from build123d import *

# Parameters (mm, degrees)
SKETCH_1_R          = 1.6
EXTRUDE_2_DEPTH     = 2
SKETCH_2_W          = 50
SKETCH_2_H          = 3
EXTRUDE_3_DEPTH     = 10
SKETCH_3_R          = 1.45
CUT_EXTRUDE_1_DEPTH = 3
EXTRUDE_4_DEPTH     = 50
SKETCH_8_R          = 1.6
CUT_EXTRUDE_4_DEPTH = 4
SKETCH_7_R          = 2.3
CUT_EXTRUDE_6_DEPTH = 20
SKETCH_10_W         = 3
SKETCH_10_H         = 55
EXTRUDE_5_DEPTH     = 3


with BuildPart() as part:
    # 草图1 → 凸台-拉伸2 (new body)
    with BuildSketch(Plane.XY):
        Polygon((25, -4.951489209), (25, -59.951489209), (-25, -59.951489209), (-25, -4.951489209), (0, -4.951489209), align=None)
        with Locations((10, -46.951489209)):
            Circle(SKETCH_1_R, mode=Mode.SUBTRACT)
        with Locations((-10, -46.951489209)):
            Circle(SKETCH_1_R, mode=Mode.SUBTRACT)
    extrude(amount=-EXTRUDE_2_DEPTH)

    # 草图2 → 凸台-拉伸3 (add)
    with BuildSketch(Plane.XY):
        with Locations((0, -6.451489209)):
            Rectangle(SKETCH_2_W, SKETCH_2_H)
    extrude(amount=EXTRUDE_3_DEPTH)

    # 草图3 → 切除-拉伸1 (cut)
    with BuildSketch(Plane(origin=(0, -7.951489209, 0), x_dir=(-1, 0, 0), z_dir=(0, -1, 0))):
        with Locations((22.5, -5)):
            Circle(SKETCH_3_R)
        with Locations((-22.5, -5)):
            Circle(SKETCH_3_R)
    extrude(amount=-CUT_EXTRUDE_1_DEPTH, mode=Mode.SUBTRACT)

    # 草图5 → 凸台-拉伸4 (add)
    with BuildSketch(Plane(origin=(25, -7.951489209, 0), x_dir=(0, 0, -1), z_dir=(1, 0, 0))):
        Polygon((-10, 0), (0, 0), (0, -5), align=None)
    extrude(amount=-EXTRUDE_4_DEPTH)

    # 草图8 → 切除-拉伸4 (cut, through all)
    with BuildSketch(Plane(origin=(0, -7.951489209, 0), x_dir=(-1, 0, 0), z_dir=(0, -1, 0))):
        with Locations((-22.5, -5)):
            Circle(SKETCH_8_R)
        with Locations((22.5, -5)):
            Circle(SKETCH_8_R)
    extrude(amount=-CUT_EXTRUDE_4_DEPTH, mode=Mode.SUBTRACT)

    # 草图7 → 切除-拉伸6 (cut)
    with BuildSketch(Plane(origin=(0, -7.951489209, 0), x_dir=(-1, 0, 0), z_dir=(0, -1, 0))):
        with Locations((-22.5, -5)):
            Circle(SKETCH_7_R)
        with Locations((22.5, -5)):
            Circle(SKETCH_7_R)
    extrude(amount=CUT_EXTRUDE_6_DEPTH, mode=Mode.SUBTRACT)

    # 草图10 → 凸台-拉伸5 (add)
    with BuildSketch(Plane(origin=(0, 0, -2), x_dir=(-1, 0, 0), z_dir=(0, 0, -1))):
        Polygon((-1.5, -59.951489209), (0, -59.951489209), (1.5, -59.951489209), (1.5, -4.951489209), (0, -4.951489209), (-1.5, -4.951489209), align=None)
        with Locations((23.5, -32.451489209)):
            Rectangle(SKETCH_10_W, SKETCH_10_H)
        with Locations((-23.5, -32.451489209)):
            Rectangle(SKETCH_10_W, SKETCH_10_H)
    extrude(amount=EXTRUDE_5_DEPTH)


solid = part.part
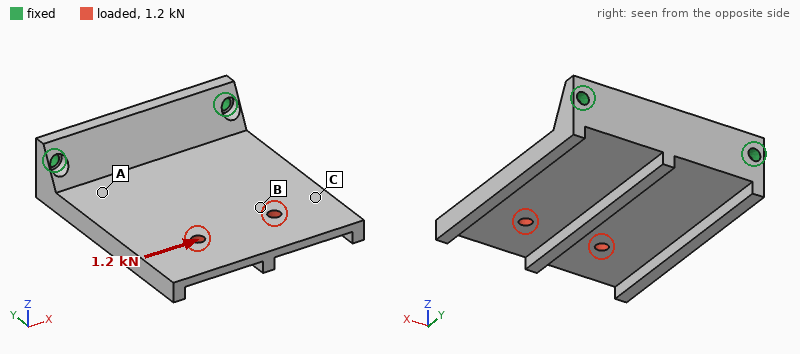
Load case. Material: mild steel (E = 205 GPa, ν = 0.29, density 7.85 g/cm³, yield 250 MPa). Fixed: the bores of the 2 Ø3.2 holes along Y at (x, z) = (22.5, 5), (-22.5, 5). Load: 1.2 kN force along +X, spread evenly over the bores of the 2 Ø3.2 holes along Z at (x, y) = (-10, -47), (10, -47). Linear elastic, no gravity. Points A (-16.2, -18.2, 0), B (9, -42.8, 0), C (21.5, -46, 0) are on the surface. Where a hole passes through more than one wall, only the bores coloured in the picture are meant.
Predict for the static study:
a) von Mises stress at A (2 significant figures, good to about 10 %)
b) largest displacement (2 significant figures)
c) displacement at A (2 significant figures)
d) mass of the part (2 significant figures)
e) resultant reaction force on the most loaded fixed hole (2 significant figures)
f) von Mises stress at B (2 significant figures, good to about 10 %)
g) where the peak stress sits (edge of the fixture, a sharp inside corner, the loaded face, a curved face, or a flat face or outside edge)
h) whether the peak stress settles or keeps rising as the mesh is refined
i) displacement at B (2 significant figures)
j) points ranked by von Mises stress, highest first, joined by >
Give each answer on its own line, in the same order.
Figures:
42 MPa
33 µm
11 µm
75 g
1.3 kN
28 MPa
edge of the fixture
keeps rising
20 µm
A > B > C
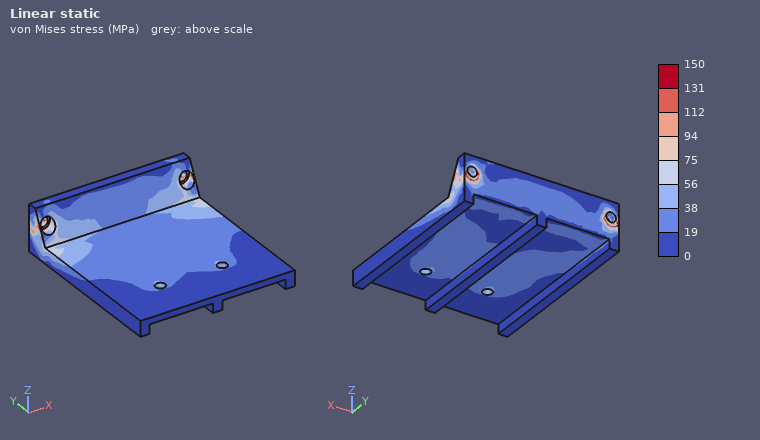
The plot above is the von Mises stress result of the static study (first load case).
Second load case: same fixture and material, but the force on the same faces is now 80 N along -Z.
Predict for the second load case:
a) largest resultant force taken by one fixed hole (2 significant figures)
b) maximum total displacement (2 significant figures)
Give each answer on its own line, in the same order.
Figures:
72 N
92 µm
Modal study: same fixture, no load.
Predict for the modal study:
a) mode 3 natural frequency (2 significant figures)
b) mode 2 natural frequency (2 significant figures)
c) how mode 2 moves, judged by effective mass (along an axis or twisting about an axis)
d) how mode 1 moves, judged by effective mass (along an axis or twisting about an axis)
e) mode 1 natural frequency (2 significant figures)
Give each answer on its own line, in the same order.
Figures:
4700 Hz
2000 Hz
twisting about Y
along Z
1100 Hz
